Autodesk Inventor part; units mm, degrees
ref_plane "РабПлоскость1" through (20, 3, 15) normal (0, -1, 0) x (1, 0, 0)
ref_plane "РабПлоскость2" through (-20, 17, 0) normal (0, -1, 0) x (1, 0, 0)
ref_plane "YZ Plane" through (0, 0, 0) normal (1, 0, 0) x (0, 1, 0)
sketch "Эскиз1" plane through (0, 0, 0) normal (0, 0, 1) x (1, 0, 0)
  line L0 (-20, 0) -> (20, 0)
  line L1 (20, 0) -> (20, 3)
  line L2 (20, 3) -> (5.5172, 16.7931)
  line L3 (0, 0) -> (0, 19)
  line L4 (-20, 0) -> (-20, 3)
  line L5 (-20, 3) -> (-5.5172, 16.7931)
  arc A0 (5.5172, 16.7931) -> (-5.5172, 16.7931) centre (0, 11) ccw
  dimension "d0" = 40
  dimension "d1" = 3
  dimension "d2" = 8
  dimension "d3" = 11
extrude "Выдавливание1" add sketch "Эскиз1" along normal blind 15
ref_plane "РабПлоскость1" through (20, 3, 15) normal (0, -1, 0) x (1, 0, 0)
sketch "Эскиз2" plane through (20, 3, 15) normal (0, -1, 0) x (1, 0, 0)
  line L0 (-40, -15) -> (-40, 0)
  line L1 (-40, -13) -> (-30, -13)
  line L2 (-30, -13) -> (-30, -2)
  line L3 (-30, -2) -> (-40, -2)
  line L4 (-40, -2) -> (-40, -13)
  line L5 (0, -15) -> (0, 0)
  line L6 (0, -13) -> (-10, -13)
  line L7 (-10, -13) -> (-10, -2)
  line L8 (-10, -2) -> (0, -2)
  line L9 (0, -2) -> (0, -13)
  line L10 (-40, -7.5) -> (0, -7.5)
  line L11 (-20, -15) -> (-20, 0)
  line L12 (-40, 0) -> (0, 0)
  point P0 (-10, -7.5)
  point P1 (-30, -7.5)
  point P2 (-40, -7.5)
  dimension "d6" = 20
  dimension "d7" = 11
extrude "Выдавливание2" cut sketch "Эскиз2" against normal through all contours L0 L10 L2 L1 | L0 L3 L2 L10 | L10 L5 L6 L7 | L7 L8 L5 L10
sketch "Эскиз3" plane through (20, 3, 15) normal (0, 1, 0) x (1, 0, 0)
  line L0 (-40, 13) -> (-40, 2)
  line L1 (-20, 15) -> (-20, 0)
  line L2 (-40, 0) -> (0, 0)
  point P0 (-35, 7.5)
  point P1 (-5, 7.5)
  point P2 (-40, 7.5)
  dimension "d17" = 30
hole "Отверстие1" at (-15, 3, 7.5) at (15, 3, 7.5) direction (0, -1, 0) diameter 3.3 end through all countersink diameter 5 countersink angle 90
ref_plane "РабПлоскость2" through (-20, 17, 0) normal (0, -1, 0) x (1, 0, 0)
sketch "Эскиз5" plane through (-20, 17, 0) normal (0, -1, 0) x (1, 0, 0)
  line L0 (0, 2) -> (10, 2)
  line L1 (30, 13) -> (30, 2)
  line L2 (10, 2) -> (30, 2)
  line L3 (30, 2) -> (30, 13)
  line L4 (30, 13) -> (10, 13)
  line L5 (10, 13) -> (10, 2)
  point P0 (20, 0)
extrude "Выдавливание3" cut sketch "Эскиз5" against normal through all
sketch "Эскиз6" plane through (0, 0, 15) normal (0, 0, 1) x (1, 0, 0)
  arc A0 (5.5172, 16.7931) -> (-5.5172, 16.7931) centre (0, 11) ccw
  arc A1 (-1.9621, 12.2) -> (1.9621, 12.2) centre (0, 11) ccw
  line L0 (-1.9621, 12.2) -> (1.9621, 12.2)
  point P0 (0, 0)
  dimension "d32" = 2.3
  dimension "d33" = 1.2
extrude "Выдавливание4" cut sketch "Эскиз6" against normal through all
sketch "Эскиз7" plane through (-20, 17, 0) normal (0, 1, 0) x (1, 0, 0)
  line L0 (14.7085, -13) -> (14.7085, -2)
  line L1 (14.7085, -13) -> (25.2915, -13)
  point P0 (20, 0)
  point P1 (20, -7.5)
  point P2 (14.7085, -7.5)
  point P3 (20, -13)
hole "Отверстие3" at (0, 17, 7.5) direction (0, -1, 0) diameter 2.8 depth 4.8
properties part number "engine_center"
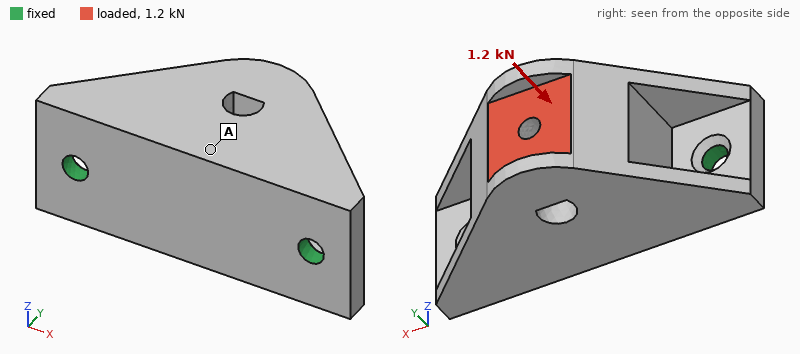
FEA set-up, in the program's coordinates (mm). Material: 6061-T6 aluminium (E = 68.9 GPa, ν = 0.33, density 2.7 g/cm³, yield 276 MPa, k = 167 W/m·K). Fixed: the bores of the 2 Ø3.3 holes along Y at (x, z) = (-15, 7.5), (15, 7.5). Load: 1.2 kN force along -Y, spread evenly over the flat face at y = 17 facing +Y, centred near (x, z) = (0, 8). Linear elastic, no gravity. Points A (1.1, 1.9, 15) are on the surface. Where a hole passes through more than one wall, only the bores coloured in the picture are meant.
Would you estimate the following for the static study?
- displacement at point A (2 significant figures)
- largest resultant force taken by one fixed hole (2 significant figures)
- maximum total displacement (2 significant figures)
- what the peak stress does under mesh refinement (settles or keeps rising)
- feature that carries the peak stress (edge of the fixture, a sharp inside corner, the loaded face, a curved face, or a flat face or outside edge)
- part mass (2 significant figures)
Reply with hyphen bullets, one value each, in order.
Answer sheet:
- 9.4 µm
- 690 N
- 10 µm
- keeps rising
- edge of the fixture
- 16 g
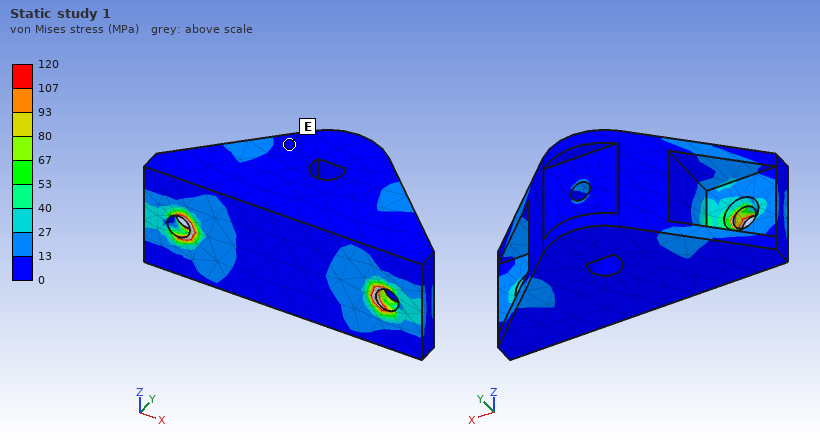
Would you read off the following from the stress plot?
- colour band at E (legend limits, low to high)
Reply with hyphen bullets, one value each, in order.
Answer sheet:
- 0 to 13 MPa
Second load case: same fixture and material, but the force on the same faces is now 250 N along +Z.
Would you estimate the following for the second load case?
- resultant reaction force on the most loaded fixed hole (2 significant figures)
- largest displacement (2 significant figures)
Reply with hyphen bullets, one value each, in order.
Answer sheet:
- 130 N
- 45 µm
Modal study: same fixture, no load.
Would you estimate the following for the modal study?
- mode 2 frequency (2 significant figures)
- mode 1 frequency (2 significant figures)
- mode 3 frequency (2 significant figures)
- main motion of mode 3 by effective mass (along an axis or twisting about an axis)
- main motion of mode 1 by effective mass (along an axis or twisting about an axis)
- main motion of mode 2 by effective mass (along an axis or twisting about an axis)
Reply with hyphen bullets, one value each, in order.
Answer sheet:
- 16 kHz
- 6000 Hz
- 20 kHz
- along X
- along Z
- along Y
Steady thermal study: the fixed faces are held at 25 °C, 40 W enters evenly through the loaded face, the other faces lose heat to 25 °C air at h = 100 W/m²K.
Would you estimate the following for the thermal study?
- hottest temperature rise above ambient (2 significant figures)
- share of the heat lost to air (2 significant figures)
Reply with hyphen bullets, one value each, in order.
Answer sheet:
- 33 K
- 11 %
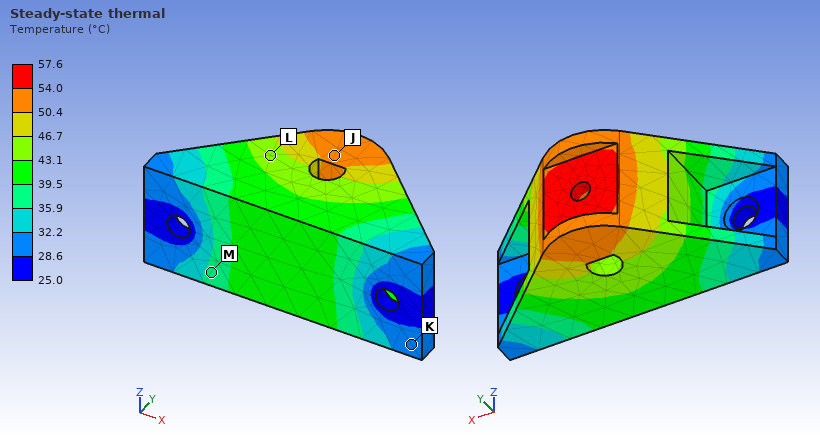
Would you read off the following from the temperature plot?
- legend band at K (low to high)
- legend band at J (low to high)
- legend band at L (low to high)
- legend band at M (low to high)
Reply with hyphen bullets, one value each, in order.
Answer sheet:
- 28.6 to 32.2 °C
- 50.4 to 54.0 °C
- 43.1 to 46.7 °C
- 35.9 to 39.5 °C
